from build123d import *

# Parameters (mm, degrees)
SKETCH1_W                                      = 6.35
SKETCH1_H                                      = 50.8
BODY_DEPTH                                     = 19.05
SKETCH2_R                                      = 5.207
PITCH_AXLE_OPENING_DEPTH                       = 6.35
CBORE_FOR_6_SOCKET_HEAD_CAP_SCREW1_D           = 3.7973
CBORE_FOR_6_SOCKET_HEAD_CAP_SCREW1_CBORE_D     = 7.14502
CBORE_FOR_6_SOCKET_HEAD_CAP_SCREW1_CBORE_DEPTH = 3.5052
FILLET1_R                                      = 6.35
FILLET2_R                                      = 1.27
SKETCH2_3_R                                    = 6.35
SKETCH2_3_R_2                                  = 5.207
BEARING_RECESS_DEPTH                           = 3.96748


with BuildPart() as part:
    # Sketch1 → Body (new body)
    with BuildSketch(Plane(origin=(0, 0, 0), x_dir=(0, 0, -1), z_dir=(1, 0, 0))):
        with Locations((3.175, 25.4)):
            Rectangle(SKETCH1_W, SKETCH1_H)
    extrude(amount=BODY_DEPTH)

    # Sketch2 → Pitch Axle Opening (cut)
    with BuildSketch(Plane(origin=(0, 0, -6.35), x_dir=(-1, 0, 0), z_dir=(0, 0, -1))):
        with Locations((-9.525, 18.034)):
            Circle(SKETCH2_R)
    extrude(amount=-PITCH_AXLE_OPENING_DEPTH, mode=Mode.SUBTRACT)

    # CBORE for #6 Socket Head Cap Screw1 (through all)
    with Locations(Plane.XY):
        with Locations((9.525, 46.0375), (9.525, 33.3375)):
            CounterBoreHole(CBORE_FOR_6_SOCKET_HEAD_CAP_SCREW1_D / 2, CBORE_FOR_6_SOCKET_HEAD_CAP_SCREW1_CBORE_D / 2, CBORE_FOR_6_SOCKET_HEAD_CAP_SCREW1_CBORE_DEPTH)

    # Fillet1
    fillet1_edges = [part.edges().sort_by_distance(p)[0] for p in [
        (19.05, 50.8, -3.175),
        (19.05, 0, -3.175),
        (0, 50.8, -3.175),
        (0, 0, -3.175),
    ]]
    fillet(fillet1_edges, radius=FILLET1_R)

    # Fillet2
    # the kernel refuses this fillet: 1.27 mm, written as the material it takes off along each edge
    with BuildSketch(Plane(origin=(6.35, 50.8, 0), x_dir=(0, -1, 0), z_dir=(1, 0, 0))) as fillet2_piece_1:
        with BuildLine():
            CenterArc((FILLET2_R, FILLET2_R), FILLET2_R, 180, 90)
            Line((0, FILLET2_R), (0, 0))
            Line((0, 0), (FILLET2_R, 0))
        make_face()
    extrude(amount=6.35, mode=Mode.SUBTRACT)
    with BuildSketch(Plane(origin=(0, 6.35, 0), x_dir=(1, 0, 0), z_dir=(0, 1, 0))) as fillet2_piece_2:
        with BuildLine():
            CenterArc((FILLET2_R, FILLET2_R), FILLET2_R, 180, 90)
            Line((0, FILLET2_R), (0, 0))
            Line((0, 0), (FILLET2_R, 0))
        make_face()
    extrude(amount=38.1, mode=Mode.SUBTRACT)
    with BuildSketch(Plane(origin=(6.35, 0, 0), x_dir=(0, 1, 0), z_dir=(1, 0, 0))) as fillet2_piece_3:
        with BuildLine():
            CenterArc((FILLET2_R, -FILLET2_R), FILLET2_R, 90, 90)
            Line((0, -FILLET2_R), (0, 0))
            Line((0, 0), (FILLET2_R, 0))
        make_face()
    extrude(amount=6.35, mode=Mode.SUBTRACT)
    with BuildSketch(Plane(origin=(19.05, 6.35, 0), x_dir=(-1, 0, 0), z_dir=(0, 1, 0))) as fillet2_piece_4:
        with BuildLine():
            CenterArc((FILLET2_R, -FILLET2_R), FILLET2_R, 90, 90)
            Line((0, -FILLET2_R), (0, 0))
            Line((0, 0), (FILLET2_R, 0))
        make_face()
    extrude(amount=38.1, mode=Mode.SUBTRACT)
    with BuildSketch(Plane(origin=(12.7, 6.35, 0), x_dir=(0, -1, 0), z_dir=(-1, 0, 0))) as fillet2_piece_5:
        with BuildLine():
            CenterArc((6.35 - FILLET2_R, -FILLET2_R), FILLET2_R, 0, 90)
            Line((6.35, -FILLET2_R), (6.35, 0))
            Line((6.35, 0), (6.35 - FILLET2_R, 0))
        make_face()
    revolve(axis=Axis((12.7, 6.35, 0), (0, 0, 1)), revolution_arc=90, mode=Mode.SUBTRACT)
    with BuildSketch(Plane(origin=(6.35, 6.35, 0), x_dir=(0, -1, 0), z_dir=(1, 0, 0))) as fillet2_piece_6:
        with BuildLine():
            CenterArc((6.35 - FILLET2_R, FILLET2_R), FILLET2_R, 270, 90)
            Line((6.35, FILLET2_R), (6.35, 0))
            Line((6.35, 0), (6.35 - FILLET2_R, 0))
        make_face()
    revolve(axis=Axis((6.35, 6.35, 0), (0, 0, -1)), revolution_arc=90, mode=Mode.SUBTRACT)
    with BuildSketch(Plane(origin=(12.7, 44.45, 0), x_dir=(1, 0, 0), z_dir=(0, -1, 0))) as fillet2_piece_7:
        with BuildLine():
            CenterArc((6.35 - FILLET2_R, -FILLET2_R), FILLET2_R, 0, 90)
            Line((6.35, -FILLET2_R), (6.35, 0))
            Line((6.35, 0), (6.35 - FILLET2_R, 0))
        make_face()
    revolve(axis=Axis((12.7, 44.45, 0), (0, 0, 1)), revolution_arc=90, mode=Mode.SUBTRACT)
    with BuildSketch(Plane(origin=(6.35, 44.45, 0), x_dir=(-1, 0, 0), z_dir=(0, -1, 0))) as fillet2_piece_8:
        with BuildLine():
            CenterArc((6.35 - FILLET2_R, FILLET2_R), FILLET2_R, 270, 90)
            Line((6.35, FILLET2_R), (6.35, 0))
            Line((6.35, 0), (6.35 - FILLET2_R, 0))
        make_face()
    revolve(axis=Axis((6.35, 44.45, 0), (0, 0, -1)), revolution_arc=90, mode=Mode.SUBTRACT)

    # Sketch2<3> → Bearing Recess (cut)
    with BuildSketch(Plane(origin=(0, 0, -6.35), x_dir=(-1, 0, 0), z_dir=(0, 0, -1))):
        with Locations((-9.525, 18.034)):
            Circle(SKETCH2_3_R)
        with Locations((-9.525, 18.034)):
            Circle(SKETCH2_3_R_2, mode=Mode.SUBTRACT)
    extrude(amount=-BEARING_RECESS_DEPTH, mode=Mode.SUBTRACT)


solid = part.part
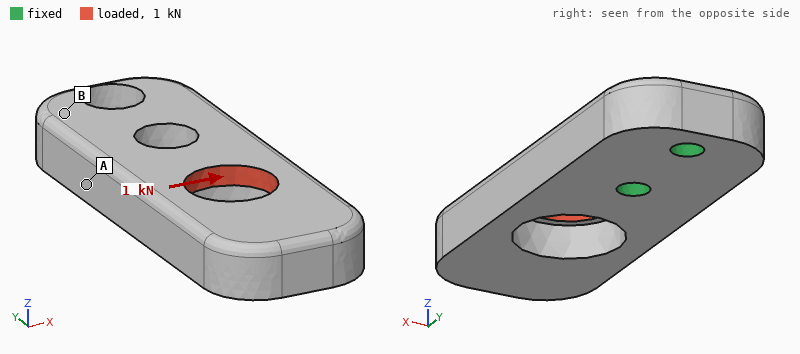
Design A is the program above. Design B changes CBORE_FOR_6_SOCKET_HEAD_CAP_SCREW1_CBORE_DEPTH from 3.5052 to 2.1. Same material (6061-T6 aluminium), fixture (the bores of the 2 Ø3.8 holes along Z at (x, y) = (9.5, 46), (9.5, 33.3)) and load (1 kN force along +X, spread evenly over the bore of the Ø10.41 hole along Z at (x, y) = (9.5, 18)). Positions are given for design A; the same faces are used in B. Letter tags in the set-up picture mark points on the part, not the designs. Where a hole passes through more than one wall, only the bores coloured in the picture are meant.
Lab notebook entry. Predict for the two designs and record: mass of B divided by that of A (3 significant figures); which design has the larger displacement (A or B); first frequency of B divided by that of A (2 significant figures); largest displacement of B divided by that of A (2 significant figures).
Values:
1.02
A
1.1
0.83
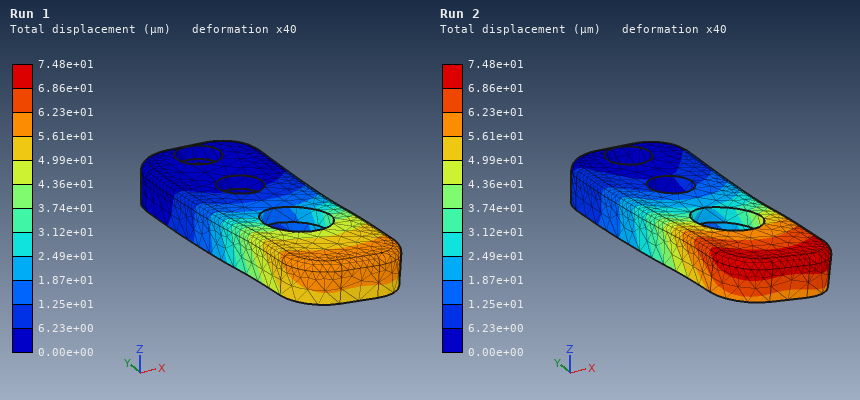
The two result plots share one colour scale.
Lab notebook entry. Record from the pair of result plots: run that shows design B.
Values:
Run 1
